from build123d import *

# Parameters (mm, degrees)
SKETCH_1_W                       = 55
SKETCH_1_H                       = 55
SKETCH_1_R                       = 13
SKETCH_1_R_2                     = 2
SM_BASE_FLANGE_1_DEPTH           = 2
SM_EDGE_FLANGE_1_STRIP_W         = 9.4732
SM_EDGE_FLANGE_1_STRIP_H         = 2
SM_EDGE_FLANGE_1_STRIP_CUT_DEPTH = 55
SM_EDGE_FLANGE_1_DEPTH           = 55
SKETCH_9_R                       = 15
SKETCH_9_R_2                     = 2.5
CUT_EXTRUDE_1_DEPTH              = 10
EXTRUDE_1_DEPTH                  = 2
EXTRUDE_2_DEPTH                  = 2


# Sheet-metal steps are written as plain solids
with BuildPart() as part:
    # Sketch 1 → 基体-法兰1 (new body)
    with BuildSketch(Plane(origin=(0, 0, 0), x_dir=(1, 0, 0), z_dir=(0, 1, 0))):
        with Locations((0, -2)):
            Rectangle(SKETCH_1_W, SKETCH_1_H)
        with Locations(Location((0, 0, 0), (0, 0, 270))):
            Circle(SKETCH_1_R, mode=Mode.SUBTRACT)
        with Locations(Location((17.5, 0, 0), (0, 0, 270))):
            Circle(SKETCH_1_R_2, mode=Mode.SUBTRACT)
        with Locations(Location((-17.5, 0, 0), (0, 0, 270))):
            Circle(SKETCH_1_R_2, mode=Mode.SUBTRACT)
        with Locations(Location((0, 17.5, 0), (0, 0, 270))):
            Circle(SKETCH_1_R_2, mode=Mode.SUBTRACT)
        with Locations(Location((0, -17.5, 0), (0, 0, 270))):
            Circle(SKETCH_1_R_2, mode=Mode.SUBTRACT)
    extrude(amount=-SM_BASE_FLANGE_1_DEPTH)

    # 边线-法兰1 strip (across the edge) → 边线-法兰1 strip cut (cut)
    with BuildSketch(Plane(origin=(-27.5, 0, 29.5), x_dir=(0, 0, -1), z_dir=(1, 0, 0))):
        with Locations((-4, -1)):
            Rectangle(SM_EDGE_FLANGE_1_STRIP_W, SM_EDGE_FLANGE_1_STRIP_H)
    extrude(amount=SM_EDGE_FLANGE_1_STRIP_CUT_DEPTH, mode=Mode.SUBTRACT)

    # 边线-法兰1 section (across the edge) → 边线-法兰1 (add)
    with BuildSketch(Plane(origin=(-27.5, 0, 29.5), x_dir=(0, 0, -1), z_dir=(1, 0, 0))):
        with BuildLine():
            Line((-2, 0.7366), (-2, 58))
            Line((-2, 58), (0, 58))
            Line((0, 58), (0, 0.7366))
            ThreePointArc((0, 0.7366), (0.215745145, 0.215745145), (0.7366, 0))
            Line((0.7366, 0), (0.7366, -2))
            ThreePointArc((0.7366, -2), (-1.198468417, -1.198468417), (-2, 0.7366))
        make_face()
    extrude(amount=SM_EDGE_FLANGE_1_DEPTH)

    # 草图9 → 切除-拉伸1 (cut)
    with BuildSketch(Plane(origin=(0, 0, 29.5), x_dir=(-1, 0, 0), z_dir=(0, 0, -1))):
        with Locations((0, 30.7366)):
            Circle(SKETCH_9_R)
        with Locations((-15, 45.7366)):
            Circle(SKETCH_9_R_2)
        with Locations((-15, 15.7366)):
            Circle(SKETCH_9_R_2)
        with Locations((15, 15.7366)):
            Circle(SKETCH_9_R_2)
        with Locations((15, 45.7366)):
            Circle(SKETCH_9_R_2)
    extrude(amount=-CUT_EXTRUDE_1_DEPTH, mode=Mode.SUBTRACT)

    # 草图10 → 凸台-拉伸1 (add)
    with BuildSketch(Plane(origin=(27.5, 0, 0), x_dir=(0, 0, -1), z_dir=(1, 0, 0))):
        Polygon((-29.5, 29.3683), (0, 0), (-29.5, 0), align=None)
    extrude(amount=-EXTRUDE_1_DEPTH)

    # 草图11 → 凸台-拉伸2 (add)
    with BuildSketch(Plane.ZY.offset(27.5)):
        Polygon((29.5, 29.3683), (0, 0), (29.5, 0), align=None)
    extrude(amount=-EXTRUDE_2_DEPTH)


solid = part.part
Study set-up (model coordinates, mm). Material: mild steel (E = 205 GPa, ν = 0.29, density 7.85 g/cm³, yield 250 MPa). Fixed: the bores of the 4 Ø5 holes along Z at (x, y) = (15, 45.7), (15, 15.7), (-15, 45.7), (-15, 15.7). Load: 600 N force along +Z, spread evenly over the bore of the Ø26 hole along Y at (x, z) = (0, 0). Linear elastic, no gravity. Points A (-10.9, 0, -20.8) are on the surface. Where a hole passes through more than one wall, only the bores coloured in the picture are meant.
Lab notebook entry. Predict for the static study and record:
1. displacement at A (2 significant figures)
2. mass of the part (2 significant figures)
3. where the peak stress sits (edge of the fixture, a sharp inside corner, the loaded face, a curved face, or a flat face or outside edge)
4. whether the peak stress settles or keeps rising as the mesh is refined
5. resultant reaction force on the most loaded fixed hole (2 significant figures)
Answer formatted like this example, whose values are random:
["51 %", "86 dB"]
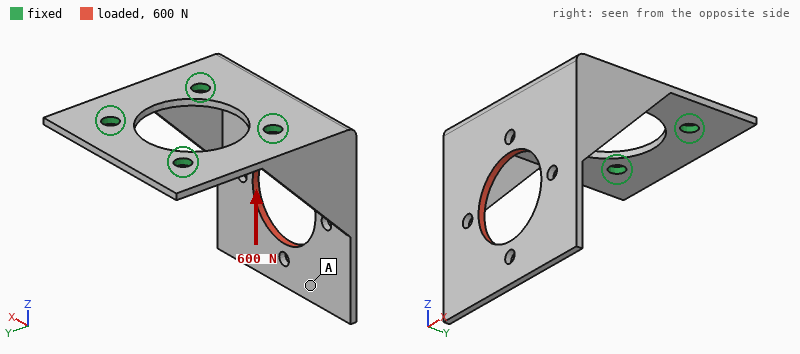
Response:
["0.16 mm", "91 g", "edge of the fixture", "keeps rising", "390 N"]
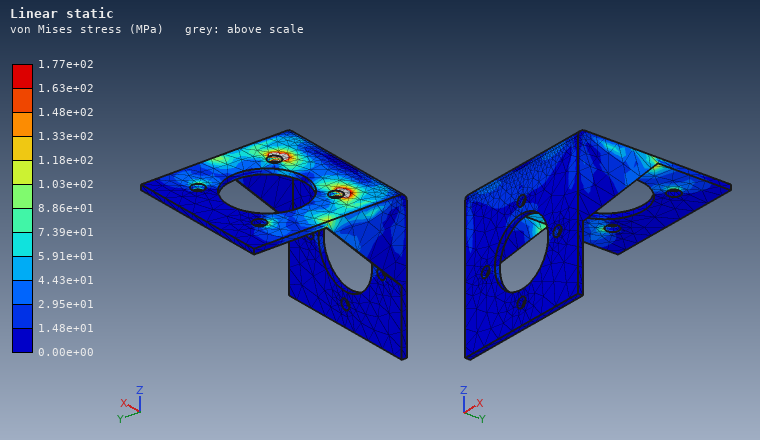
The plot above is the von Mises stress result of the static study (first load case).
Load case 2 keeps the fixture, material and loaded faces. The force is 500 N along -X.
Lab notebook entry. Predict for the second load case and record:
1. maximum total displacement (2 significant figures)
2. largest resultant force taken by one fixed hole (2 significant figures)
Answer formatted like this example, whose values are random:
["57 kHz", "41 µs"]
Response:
["0.24 mm", "570 N"]
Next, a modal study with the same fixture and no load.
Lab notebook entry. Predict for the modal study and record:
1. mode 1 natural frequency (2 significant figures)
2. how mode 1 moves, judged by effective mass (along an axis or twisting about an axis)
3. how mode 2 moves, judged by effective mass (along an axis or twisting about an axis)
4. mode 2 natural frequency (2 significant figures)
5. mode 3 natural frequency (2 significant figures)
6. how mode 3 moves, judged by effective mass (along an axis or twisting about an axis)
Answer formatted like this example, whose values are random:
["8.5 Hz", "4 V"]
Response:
["860 Hz", "along Y", "along X", "1200 Hz", "2300 Hz", "along Z"]
